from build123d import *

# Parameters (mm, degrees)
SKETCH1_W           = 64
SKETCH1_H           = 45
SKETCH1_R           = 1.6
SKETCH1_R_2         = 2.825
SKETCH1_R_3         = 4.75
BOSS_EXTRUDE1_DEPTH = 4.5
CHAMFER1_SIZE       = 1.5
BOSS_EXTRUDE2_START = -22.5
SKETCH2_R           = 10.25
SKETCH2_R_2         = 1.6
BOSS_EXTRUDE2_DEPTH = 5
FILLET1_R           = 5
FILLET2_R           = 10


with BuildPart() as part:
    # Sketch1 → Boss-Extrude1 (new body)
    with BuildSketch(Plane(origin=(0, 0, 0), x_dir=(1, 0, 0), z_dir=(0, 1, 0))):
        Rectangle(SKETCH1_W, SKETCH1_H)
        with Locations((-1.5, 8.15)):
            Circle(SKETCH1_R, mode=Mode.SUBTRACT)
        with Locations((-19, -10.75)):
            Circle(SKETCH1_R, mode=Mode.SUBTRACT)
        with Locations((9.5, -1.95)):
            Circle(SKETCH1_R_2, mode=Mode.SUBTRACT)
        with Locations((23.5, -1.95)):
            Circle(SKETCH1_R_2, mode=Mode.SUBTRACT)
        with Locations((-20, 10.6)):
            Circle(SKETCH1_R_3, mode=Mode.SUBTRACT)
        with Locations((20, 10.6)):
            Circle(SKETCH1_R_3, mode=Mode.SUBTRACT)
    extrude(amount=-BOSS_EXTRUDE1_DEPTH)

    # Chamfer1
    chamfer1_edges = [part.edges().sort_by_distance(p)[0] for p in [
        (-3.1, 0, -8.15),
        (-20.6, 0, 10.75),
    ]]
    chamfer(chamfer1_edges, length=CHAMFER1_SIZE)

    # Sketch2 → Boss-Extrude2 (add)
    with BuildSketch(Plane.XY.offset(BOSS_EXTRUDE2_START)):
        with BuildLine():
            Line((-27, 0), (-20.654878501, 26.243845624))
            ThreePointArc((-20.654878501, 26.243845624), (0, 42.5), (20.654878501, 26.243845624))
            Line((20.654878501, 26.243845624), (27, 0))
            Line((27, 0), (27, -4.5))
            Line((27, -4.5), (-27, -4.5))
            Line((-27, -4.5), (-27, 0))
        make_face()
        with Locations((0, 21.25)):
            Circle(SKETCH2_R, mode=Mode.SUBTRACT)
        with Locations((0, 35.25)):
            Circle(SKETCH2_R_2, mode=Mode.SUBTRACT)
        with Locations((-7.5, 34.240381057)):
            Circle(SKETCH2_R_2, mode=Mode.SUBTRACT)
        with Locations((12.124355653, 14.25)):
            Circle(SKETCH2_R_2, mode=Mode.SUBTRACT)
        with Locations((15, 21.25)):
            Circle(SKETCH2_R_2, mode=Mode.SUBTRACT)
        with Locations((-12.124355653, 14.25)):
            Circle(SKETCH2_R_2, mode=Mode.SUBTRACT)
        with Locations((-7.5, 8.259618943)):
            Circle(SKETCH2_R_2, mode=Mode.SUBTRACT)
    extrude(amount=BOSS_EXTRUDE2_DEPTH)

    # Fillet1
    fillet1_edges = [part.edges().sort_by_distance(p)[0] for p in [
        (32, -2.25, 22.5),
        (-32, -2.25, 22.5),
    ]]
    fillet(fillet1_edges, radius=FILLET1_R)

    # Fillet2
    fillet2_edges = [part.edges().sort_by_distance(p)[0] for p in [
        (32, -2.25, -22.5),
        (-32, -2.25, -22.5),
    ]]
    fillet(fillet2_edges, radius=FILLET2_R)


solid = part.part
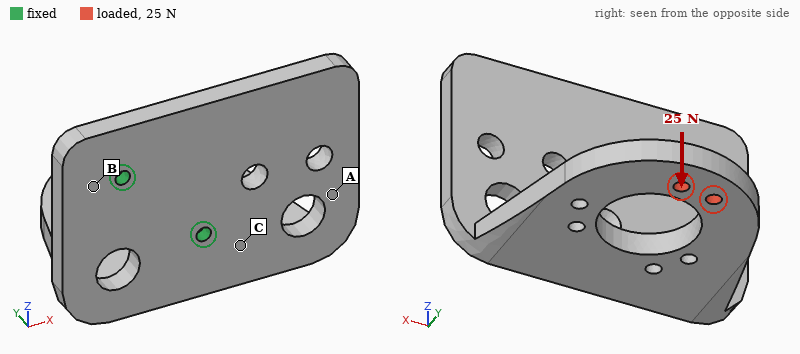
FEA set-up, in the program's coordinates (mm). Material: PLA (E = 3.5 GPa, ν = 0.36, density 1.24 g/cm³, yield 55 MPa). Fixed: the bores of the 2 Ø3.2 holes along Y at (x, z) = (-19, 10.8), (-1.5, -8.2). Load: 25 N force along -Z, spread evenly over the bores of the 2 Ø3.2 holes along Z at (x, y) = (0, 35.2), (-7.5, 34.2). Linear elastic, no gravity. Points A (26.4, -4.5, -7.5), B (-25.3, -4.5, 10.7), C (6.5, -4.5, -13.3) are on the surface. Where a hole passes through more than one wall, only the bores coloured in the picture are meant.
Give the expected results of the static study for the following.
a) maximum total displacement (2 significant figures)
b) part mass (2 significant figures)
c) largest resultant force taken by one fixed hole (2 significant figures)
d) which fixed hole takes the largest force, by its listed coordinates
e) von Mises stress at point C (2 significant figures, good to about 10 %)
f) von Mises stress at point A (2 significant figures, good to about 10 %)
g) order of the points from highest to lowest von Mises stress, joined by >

1.0 mm
23 g
26 N
(-19, 10.8)
5.1 MPa
2.8 MPa
C > A > B
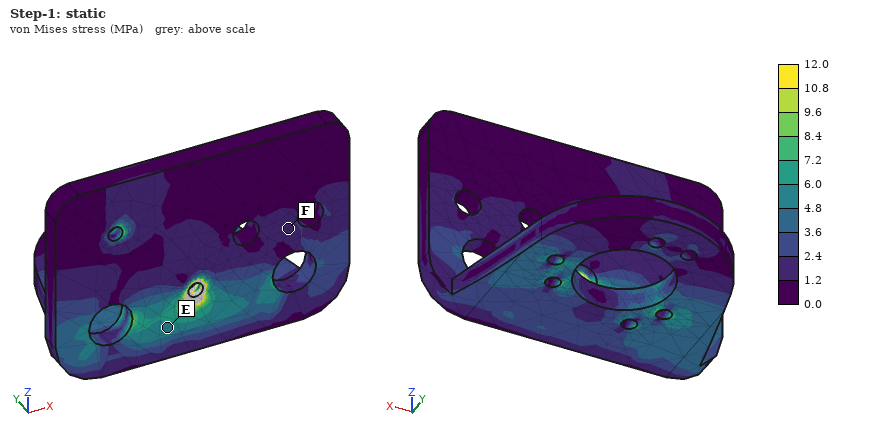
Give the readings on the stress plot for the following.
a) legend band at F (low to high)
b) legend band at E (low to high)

1.2 to 2.4 MPa
4.8 to 6.0 MPa
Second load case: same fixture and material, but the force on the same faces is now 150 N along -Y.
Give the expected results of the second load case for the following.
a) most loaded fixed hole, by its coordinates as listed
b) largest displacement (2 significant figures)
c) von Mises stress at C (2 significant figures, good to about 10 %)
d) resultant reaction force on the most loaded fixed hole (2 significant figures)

(-1.5, -8.2)
0.89 mm
5.8 MPa
170 N
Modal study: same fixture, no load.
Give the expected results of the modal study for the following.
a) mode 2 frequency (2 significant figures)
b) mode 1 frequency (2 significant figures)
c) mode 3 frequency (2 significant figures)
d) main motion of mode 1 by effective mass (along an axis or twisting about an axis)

610 Hz
470 Hz
1000 Hz
along Z
